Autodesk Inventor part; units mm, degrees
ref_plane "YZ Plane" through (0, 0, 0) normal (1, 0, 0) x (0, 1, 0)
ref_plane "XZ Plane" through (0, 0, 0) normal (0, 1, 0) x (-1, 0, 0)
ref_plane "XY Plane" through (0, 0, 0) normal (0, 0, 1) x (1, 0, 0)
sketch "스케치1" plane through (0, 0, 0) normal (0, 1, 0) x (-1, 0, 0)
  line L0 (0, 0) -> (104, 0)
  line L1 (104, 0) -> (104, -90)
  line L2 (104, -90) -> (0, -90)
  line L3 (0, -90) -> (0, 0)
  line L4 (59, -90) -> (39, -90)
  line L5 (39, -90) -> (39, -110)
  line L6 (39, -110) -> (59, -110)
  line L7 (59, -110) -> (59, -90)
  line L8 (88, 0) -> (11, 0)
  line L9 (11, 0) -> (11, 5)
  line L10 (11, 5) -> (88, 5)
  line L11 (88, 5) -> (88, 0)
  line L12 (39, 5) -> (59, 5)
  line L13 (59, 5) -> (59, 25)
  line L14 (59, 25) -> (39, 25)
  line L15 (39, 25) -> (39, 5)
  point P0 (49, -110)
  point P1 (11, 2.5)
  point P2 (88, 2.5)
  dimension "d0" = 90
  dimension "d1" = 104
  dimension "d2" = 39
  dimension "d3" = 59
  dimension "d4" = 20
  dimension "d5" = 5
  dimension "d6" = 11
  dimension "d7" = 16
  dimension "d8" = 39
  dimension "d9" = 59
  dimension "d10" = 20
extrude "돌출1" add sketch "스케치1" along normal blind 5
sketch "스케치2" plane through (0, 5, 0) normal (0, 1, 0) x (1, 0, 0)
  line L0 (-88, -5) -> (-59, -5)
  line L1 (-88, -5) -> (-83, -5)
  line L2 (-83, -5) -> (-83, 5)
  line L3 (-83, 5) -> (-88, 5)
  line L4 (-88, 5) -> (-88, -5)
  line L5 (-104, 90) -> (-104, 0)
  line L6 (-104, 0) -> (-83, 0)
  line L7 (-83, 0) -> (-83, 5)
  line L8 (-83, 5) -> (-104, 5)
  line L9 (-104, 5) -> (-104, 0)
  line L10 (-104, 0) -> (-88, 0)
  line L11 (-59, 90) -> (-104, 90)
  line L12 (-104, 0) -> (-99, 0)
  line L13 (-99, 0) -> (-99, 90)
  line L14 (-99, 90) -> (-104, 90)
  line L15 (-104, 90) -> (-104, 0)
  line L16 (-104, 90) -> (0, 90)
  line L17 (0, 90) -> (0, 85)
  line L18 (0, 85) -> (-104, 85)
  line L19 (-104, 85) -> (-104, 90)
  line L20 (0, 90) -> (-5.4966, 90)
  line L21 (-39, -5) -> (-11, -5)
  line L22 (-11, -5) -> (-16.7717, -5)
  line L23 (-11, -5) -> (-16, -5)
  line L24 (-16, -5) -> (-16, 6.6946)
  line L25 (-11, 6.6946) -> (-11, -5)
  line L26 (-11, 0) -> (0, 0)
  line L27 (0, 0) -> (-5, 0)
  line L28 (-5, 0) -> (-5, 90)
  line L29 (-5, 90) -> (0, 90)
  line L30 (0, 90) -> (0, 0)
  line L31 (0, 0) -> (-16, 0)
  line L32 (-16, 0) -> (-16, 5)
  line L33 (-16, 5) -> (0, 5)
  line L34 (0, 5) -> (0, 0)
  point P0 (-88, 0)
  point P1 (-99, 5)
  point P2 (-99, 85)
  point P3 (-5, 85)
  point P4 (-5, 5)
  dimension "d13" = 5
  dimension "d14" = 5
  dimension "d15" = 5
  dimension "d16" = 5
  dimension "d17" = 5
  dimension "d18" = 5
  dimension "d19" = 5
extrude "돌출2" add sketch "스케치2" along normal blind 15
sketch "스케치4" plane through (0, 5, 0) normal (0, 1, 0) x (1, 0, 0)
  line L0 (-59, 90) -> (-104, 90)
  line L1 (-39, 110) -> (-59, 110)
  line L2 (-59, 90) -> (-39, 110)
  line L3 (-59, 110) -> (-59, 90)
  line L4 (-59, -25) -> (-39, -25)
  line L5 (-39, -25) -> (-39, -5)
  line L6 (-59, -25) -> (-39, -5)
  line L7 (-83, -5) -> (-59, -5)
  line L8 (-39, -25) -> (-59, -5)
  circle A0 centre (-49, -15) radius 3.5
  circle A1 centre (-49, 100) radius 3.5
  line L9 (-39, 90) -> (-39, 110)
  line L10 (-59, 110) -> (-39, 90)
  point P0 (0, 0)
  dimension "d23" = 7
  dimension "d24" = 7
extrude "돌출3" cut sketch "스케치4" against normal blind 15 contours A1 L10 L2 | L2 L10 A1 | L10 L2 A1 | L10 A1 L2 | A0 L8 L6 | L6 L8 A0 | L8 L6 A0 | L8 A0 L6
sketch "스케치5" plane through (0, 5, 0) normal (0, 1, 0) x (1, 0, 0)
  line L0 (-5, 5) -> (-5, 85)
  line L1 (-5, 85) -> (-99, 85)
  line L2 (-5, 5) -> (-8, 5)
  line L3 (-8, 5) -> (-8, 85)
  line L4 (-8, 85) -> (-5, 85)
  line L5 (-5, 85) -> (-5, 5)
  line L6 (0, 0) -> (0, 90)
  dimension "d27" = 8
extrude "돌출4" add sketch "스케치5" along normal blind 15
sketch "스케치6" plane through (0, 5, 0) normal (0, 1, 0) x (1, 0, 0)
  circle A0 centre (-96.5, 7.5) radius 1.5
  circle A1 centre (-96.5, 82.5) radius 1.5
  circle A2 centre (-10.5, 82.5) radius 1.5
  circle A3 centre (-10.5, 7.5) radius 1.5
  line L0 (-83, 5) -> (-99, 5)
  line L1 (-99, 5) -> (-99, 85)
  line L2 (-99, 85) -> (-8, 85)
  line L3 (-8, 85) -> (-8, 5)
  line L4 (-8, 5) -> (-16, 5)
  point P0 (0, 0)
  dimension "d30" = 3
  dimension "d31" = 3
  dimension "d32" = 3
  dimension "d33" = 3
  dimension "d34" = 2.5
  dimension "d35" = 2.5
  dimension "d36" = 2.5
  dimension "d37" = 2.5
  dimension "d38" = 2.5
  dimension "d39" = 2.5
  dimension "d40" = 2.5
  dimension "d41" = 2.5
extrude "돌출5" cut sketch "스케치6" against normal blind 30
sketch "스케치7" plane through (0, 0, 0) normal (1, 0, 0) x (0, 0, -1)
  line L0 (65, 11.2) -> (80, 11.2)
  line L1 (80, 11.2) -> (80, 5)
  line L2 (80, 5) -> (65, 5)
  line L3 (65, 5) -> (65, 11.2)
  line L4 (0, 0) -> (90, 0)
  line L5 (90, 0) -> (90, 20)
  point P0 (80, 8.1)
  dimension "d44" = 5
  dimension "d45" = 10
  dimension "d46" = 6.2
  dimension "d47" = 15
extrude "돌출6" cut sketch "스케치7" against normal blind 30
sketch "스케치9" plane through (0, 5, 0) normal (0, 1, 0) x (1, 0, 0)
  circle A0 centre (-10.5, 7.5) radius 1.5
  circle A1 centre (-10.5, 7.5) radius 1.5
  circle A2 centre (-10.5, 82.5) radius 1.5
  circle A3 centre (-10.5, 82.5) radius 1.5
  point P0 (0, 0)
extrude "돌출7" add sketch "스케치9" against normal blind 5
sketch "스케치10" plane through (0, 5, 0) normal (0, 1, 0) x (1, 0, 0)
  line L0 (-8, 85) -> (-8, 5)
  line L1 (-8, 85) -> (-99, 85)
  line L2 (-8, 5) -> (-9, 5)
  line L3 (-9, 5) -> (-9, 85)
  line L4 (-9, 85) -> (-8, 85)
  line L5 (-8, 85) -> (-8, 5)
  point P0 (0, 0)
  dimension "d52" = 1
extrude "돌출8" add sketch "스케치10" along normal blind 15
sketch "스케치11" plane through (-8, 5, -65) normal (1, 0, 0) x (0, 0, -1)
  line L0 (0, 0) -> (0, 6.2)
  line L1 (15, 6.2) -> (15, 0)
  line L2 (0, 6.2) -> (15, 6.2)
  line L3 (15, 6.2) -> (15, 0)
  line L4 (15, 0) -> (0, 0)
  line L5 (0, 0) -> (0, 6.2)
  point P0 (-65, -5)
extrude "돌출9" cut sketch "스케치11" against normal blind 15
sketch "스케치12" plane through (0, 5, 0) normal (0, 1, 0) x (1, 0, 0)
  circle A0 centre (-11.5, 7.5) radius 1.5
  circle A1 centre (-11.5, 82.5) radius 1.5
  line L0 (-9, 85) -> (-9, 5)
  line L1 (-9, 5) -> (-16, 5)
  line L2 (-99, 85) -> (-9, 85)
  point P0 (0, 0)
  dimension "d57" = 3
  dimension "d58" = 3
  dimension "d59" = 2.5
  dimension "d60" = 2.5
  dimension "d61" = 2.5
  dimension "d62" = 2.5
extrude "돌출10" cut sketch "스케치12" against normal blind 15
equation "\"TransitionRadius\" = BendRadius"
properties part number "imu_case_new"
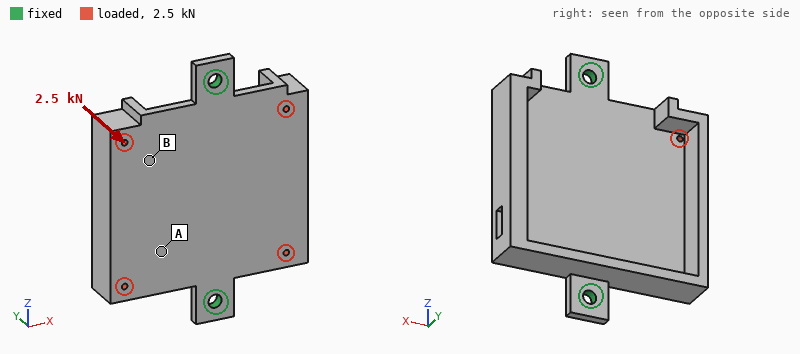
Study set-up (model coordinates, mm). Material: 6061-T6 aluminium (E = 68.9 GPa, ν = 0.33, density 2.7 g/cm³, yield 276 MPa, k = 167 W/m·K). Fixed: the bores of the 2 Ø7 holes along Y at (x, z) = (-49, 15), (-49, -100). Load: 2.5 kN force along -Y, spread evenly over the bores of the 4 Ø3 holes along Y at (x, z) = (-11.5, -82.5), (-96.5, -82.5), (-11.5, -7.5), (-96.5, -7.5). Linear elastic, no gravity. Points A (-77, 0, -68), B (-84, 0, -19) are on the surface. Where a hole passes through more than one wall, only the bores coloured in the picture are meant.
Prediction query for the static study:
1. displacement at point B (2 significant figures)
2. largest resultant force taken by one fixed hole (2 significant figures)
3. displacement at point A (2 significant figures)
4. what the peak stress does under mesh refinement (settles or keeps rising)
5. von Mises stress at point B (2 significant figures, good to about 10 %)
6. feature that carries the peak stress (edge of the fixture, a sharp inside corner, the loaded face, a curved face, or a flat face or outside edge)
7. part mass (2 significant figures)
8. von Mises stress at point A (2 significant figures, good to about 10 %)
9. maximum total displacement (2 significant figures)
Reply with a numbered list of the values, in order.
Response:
1. 0.42 mm
2. 1.3 kN
3. 0.24 mm
4. keeps rising
5. 46 MPa
6. edge of the fixture
7. 210 g
8. 22 MPa
9. 0.83 mm
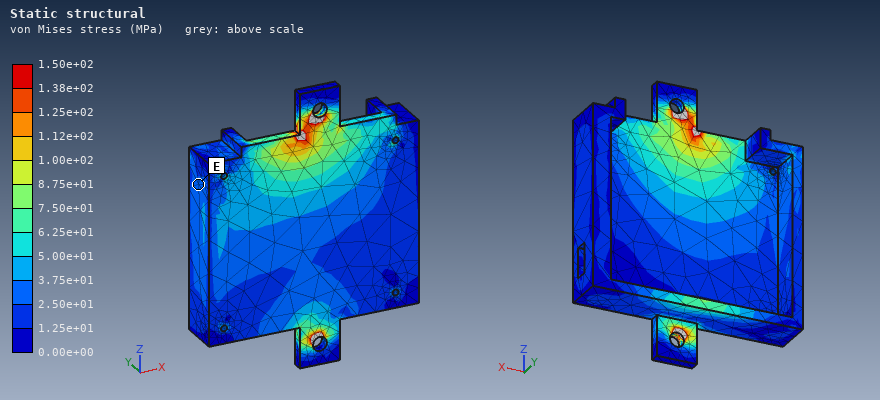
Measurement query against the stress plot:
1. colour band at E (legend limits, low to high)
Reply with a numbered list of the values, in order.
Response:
1. 2.50e+01 to 3.75e+01 MPa
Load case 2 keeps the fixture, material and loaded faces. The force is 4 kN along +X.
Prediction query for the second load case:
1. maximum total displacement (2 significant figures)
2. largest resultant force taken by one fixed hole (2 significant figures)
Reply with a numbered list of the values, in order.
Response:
1. 24 µm
2. 2.1 kN
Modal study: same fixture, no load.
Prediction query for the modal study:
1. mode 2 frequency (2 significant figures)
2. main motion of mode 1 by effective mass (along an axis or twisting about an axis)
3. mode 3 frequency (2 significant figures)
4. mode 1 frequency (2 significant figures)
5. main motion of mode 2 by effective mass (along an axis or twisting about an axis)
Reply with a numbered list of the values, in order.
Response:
1. 1200 Hz
2. twisting about Z
3. 1800 Hz
4. 610 Hz
5. along Y
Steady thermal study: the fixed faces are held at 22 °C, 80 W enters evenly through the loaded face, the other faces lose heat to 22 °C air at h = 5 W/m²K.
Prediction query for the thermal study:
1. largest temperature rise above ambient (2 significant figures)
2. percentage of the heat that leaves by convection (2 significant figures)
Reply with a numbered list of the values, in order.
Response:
1. 60 K
2. 8.4 %
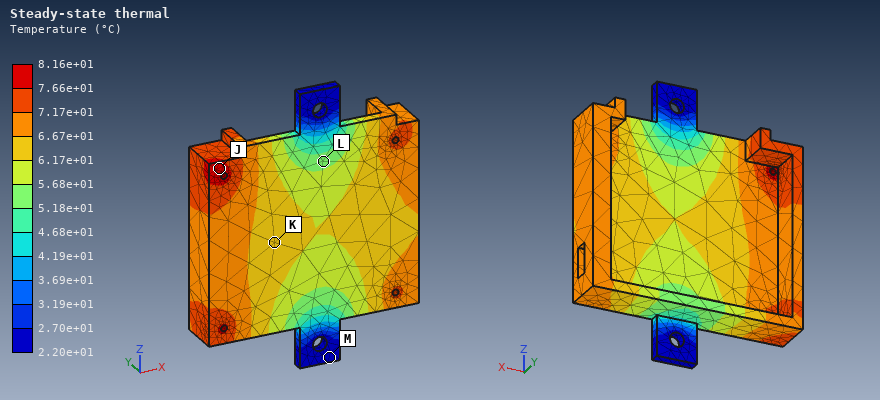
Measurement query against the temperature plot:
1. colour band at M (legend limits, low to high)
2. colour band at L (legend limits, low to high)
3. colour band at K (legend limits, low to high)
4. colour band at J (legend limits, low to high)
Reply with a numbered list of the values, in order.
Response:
1. 2.20e+01 to 2.70e+01 °C
2. 5.18e+01 to 5.68e+01 °C
3. 6.17e+01 to 6.67e+01 °C
4. 7.66e+01 to 8.16e+01 °C
